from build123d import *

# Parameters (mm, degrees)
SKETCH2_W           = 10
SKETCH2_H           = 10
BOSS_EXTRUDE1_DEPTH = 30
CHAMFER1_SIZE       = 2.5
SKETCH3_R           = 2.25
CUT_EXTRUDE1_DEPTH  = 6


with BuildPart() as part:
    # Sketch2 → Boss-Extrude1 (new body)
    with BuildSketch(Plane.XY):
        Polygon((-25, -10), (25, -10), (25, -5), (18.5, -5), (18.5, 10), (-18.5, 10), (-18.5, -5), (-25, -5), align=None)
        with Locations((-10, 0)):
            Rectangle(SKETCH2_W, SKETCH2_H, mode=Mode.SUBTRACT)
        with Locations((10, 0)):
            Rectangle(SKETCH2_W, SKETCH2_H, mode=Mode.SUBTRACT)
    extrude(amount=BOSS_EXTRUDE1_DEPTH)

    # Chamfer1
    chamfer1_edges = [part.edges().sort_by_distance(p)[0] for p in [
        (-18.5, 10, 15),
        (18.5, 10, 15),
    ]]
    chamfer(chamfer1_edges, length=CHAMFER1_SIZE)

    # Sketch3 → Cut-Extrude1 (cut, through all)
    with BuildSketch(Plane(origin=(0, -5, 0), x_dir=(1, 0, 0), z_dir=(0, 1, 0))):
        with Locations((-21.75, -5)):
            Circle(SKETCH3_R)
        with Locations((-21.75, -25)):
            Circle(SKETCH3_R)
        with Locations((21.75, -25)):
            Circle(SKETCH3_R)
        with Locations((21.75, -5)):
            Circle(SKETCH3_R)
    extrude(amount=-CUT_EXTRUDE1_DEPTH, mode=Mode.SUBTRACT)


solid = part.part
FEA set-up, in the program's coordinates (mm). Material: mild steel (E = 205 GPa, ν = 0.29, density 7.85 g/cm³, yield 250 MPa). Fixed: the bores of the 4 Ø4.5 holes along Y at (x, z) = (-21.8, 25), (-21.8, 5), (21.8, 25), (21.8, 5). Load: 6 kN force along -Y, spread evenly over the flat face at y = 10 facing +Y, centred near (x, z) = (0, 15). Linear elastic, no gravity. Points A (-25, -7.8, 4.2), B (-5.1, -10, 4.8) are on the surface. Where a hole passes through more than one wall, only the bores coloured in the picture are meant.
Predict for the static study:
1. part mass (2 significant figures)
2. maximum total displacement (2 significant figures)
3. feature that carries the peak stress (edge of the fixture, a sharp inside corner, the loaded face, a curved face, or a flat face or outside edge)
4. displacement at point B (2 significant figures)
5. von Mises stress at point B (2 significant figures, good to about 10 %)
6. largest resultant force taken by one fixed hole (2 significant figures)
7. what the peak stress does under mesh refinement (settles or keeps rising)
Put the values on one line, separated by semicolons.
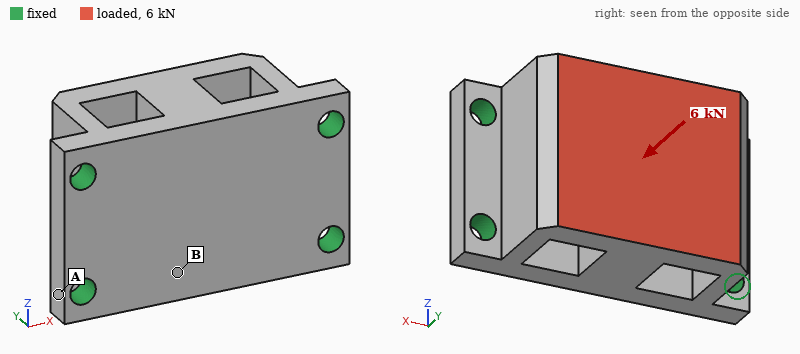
140 g; 10 µm; edge of the fixture; 9.1 µm; 41 MPa; 1.6 kN; keeps rising
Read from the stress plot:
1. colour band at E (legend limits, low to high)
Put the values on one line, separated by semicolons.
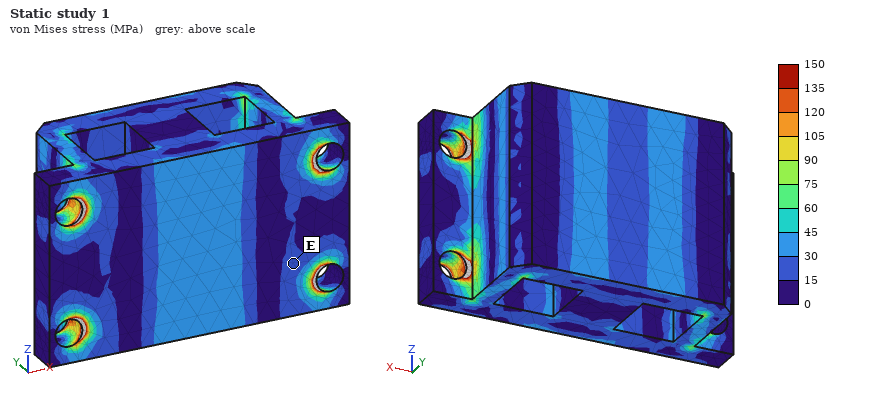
15 to 30 MPa
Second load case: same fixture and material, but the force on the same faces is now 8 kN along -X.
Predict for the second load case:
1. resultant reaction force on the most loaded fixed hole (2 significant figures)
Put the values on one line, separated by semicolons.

2.8 kN
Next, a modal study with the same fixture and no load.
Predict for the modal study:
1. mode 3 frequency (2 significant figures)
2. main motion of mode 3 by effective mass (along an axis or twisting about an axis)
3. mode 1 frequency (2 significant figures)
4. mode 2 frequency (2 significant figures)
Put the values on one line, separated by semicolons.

15 kHz; along X; 13 kHz; 13 kHz
